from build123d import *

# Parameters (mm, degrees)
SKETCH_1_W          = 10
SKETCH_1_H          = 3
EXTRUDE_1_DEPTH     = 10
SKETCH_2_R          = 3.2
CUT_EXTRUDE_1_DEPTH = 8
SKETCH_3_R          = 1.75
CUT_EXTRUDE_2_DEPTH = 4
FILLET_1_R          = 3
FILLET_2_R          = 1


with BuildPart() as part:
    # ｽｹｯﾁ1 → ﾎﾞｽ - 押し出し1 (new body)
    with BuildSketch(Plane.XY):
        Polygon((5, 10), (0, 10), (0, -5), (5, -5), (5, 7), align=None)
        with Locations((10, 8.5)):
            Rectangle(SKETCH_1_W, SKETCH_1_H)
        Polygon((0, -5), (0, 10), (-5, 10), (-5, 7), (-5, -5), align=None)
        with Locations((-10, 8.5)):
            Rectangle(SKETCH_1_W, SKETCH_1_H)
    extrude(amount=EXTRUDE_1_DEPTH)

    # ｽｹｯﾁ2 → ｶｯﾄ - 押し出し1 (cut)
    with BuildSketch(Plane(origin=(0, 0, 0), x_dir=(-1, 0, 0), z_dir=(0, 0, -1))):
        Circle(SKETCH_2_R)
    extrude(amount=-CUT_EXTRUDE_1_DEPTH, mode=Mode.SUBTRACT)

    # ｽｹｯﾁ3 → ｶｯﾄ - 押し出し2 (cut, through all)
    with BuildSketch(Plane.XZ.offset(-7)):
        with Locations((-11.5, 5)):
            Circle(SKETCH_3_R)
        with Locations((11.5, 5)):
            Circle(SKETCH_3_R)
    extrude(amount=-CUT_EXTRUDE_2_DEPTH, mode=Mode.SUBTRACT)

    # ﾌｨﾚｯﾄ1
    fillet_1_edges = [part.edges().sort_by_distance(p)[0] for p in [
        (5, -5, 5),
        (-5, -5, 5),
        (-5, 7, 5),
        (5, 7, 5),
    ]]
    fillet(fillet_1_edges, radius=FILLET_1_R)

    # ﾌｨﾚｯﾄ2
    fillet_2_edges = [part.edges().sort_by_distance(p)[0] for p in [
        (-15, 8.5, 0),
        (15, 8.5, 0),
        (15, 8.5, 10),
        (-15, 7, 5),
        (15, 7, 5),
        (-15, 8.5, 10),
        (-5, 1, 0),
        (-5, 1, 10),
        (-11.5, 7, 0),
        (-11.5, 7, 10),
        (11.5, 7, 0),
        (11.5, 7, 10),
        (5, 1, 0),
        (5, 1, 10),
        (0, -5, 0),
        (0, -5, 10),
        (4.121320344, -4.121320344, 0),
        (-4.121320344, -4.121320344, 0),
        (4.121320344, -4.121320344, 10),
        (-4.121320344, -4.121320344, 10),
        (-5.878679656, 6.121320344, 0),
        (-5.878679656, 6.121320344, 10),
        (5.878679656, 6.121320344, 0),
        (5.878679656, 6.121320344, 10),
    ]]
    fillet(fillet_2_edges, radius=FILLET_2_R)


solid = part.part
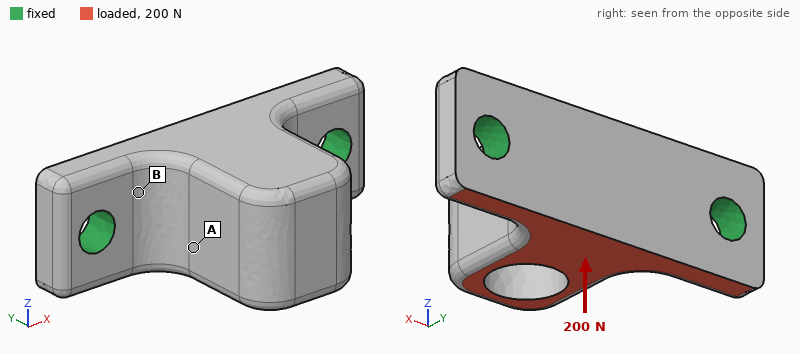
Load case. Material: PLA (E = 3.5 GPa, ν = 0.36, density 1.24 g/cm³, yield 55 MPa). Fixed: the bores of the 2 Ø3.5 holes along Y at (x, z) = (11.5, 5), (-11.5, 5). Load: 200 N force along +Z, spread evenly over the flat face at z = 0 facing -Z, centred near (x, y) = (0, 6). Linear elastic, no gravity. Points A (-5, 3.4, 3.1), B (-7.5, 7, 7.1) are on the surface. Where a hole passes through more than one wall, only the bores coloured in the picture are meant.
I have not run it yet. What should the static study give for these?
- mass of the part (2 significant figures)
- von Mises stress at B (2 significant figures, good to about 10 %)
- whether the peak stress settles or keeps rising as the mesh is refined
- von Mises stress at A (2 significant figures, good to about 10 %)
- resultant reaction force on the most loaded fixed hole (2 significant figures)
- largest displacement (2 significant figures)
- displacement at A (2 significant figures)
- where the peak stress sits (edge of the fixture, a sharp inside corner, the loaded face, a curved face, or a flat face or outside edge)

2.2 g
17 MPa
keeps rising
3.3 MPa
100 N
0.19 mm
0.083 mm
edge of the fixture
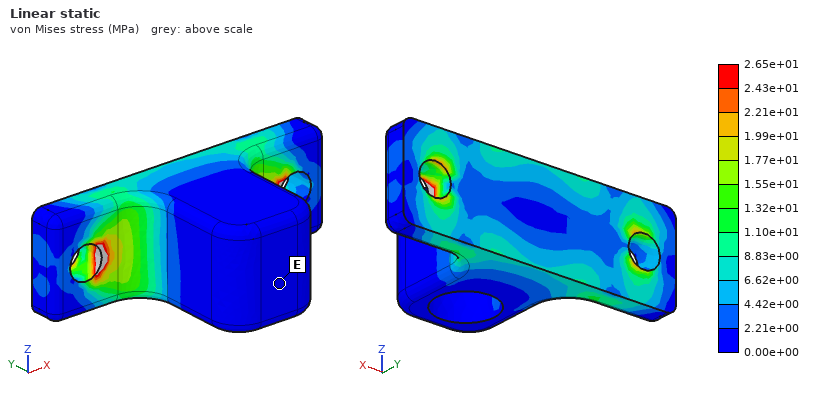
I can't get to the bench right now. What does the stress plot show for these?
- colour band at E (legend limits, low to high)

0.00e+00 to 2.21e+00 MPa
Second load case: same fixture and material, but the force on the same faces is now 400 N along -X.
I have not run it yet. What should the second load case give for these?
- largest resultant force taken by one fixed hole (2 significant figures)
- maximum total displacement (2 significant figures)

220 N
0.10 mm
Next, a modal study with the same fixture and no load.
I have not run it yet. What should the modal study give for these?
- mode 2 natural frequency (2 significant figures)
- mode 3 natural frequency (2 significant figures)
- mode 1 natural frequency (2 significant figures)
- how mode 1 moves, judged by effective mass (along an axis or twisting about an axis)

8200 Hz
8400 Hz
3600 Hz
along Z
